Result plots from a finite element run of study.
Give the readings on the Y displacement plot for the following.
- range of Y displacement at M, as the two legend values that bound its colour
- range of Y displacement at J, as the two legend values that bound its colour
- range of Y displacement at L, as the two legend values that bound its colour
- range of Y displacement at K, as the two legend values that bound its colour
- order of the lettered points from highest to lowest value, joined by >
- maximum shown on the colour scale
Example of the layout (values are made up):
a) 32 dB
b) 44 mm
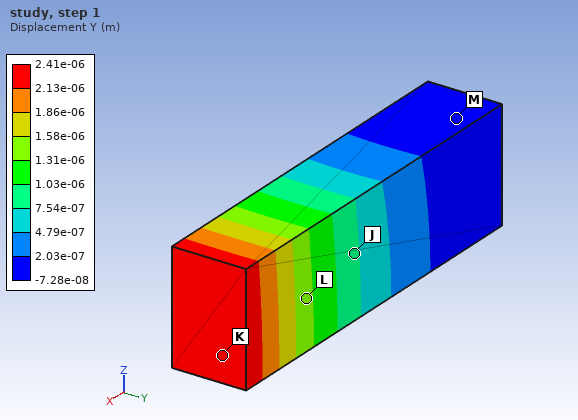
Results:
a) -7.28e-08 to 2.03e-07 m
b) 7.54e-07 to 1.03e-06 m
c) 1.31e-06 to 1.58e-06 m
d) 2.13e-06 to 2.41e-06 m
e) K > L > J > M
f) 2.41e-06 m
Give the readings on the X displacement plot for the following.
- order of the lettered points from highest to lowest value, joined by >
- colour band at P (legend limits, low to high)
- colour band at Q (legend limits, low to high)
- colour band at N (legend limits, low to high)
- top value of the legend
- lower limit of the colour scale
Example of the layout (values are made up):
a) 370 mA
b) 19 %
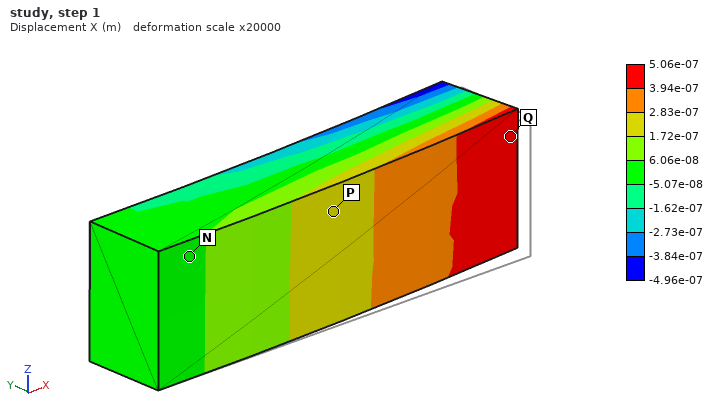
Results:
a) Q > P > N
b) 1.72e-07 to 2.83e-07 m
c) 3.94e-07 to 5.06e-07 m
d) -5.07e-08 to 6.06e-08 m
e) 5.06e-07 m
f) -4.96e-07 m
